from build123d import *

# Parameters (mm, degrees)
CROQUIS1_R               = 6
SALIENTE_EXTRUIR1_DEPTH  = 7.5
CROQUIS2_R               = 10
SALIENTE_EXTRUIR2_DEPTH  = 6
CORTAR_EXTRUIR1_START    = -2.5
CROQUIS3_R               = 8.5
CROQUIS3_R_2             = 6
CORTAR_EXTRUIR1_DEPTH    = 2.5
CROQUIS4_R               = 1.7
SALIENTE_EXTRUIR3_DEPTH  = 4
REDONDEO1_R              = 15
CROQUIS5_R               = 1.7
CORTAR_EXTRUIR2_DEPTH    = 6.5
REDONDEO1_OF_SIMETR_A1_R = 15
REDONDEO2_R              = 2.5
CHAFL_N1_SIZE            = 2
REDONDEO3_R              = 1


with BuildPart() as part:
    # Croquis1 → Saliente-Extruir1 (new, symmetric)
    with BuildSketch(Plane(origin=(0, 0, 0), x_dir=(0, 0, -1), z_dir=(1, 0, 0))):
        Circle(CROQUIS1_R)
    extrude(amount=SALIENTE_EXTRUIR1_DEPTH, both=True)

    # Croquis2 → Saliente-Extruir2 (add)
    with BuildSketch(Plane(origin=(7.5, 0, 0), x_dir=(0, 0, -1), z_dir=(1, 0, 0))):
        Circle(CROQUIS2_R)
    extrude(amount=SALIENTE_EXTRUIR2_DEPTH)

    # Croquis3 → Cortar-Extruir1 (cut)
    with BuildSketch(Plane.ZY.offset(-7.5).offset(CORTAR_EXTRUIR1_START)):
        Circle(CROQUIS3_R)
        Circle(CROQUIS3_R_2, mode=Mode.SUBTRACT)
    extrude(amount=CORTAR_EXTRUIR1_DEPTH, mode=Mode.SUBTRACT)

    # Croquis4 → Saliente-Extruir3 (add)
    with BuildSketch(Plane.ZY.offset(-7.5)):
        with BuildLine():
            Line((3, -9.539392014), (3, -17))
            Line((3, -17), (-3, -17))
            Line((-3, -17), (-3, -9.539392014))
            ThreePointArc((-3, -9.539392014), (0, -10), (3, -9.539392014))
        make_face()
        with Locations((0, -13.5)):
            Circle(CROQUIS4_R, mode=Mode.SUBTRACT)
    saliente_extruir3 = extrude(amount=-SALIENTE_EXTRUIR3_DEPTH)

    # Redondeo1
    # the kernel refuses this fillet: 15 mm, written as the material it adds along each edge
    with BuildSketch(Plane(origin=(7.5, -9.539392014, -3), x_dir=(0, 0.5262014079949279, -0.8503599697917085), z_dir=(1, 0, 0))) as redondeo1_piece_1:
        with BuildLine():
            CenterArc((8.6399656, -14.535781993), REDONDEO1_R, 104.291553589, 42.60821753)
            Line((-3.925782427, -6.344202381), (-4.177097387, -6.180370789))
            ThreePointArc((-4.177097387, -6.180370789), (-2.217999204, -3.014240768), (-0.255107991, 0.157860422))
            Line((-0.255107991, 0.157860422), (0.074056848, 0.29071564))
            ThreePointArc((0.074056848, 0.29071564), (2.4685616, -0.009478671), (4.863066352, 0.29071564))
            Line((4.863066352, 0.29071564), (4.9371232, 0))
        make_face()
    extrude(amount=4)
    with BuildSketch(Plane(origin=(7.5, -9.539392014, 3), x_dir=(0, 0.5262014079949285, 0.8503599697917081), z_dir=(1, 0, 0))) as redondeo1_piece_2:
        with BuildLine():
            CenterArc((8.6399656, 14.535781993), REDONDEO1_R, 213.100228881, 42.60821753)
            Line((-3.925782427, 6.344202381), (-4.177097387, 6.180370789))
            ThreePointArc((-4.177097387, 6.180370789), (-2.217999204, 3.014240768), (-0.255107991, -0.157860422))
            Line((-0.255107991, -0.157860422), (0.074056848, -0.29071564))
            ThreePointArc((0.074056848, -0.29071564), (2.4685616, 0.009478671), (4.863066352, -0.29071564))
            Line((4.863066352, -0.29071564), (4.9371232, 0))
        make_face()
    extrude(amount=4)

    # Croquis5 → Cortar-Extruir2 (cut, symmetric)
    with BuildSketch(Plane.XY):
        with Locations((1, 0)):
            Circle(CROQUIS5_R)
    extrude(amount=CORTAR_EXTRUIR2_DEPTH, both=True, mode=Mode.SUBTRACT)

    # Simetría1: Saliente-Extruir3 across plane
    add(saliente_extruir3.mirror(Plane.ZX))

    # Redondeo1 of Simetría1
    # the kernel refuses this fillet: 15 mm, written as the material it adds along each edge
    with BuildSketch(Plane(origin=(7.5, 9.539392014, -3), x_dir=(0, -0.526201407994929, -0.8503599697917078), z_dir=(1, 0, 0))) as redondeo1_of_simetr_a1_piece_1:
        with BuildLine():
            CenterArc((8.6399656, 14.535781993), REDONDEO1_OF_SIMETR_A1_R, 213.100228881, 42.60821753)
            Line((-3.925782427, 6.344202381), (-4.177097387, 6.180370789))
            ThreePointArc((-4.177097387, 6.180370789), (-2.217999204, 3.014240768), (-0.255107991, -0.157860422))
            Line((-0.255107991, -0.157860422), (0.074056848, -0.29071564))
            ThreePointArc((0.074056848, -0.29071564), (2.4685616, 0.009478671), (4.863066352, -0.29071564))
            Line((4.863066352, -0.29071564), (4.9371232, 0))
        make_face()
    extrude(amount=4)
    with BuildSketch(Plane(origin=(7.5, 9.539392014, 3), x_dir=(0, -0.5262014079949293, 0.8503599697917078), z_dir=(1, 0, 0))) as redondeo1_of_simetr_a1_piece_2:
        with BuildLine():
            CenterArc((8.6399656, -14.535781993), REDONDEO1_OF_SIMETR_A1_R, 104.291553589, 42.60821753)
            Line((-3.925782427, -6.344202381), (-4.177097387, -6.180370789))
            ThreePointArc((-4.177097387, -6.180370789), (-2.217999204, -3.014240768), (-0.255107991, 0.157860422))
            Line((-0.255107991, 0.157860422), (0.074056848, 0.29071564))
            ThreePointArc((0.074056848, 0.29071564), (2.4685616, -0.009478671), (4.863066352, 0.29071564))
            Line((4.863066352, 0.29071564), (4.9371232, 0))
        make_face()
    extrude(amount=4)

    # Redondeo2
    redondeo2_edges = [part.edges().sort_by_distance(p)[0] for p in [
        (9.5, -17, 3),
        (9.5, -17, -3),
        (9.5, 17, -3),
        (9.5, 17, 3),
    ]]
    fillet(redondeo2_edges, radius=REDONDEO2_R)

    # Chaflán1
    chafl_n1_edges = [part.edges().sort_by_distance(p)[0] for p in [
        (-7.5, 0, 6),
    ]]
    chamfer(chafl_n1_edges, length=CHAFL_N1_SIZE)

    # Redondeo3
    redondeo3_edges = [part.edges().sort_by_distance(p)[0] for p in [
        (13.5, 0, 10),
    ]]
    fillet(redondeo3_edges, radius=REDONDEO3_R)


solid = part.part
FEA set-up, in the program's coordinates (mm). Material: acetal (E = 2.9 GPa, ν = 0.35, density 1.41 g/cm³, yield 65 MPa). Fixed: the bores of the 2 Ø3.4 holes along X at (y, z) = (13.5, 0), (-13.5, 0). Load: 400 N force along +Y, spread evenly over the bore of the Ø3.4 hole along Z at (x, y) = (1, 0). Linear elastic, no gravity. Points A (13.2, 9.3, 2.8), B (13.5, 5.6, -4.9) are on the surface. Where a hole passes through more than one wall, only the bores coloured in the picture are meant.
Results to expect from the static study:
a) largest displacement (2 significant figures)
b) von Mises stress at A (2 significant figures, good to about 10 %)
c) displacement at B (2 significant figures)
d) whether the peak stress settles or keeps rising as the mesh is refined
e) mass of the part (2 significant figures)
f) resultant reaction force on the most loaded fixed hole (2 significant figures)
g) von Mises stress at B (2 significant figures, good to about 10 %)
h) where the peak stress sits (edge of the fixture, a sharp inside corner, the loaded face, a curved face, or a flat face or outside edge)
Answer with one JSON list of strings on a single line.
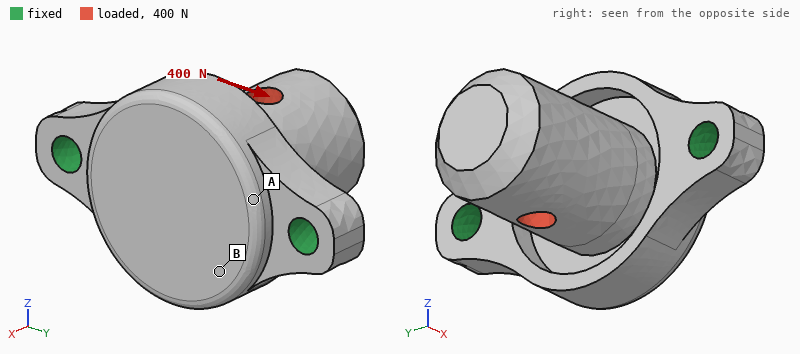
["0.47 mm", "6.7 MPa", "0.071 mm", "keeps rising", "4.9 g", "280 N", "17 MPa", "edge of the fixture"]
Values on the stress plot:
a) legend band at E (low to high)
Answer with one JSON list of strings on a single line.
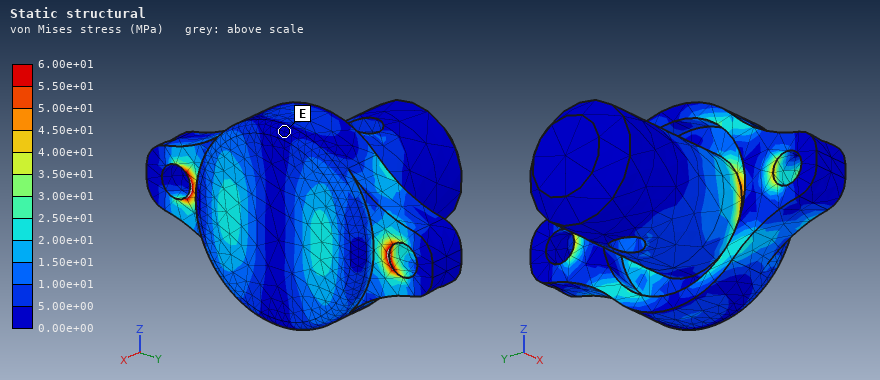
["0.00e+00 to 5.00e+00 MPa"]
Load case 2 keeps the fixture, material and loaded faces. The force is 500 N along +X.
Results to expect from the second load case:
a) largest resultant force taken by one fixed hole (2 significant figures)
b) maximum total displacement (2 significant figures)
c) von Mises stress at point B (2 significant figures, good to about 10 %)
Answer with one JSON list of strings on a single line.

["320 N", "0.16 mm", "15 MPa"]
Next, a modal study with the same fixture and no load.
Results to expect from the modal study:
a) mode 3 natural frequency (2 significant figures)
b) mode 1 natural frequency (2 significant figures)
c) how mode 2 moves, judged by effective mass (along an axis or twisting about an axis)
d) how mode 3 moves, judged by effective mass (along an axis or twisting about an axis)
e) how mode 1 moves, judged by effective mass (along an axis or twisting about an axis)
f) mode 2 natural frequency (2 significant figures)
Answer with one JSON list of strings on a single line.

["4600 Hz", "2000 Hz", "along Y", "along X", "along Z", "3500 Hz"]
